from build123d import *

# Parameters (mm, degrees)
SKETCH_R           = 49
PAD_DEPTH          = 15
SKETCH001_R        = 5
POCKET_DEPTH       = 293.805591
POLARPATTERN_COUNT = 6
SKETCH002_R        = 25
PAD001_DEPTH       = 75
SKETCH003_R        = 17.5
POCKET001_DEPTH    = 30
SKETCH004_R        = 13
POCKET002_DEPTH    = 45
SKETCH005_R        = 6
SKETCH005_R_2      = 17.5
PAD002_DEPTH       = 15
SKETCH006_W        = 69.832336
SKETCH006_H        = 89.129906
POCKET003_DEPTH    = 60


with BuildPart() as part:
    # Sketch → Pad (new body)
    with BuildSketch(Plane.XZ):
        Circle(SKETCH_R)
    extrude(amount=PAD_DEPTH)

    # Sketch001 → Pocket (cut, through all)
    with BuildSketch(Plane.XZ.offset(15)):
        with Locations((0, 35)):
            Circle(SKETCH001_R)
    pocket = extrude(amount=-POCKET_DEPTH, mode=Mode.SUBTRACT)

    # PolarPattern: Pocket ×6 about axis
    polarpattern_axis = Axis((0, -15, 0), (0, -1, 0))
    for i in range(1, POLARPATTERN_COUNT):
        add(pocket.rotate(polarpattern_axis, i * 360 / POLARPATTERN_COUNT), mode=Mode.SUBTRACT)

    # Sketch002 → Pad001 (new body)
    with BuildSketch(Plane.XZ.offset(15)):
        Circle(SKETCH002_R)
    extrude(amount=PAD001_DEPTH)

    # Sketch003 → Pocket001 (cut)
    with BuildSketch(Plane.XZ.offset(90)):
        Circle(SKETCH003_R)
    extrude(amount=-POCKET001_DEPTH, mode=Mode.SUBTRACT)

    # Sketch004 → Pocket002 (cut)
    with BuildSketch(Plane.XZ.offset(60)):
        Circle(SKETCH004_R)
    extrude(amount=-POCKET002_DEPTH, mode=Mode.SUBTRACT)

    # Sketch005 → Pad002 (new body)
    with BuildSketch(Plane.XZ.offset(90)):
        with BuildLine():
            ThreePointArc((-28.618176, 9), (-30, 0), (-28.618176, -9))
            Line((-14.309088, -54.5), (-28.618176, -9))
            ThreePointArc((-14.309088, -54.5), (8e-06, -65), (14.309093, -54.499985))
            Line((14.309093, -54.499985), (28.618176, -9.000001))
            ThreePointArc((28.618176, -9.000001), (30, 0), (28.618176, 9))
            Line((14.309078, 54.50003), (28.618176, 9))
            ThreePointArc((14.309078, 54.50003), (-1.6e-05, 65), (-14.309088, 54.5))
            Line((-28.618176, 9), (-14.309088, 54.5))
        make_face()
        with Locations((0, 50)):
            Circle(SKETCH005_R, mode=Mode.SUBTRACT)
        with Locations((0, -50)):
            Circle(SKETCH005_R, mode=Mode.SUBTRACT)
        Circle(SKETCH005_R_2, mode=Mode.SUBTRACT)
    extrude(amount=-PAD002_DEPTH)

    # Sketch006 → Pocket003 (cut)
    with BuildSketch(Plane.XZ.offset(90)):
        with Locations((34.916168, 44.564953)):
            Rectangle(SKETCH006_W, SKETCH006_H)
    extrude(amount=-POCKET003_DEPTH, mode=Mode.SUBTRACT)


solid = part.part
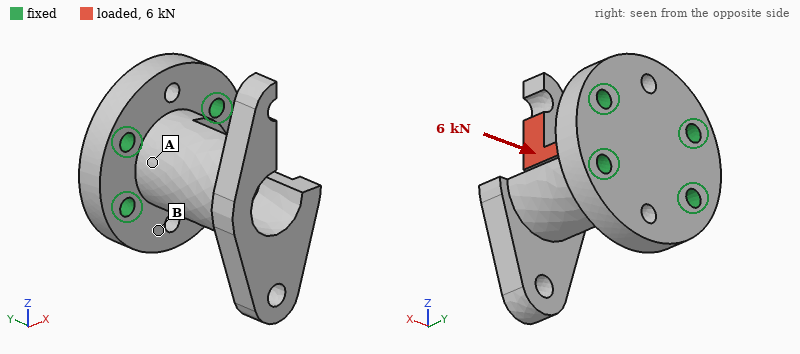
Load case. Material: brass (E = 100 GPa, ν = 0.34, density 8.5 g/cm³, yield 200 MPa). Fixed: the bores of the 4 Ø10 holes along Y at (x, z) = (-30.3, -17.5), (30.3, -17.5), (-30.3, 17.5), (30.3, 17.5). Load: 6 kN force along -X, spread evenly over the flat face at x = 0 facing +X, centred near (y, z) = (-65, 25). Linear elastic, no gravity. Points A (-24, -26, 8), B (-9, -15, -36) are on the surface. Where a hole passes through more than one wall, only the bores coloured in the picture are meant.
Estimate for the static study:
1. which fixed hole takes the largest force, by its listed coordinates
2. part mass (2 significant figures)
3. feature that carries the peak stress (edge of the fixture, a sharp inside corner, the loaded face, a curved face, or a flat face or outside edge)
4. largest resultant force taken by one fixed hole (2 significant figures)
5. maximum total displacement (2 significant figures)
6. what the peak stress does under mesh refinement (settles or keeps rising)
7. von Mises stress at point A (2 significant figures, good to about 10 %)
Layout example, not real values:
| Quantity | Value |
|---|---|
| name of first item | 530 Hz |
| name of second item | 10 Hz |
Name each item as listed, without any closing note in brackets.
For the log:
| Quantity | Value |
|---|---|
| which fixed hole takes the largest force, by its listed coordinates | (30.3, 17.5) |
| part mass | 1.9 kg |
| feature that carries the peak stress | a sharp inside corner |
| largest resultant force taken by one fixed hole | 4.4 kN |
| maximum total displacement | 0.53 mm |
| what the peak stress does under mesh refinement | keeps rising |
| von Mises stress at point A | 67 MPa |
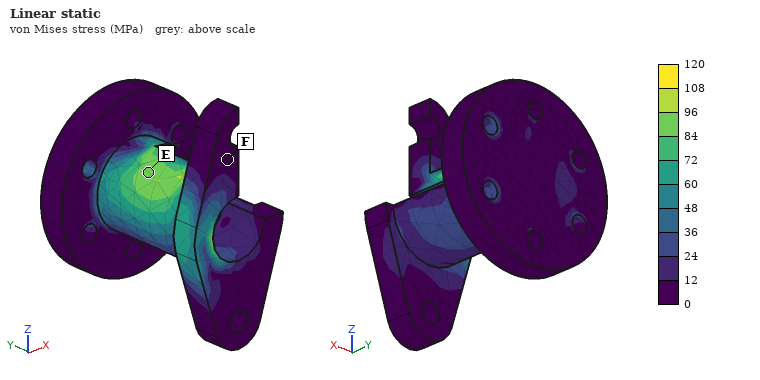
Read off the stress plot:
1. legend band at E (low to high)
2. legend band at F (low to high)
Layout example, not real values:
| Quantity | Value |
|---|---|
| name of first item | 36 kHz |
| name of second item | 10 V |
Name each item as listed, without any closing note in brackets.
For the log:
| Quantity | Value |
|---|---|
| legend band at E | 84 to 96 MPa |
| legend band at F | 0 to 12 MPa |
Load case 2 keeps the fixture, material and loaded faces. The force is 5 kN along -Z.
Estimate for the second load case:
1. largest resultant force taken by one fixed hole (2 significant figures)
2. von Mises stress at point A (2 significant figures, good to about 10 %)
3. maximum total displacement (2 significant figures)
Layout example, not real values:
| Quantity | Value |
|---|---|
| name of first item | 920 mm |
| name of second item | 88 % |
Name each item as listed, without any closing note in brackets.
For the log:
| Quantity | Value |
|---|---|
| largest resultant force taken by one fixed hole | 4.4 kN |
| von Mises stress at point A | 24 MPa |
| maximum total displacement | 0.33 mm |
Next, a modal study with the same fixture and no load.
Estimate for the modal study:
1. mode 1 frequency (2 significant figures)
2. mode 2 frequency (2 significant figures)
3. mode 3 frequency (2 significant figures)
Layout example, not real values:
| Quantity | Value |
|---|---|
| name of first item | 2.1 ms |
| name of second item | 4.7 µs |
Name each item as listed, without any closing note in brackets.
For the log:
| Quantity | Value |
|---|---|
| mode 1 frequency | 1200 Hz |
| mode 2 frequency | 1700 Hz |
| mode 3 frequency | 2300 Hz |
